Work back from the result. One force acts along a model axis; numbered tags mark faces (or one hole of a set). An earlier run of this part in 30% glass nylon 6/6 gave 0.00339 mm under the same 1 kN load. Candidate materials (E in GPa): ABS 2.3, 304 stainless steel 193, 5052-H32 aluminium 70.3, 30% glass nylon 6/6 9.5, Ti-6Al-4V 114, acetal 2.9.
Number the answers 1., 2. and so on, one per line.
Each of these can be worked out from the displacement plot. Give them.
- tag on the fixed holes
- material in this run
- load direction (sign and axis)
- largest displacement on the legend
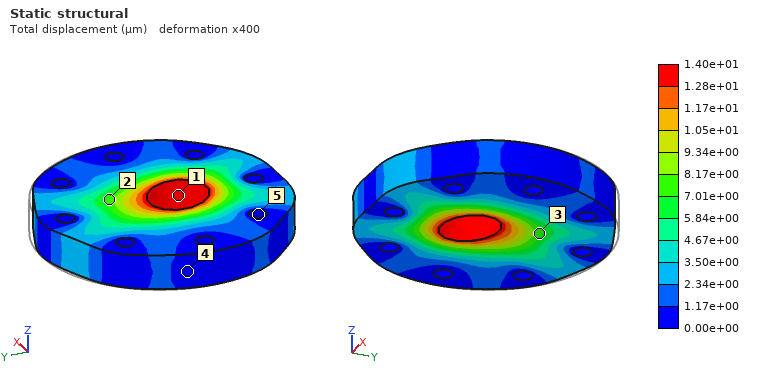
1. 5
2. ABS
3. -Y
4. 1.40e+01 µm
